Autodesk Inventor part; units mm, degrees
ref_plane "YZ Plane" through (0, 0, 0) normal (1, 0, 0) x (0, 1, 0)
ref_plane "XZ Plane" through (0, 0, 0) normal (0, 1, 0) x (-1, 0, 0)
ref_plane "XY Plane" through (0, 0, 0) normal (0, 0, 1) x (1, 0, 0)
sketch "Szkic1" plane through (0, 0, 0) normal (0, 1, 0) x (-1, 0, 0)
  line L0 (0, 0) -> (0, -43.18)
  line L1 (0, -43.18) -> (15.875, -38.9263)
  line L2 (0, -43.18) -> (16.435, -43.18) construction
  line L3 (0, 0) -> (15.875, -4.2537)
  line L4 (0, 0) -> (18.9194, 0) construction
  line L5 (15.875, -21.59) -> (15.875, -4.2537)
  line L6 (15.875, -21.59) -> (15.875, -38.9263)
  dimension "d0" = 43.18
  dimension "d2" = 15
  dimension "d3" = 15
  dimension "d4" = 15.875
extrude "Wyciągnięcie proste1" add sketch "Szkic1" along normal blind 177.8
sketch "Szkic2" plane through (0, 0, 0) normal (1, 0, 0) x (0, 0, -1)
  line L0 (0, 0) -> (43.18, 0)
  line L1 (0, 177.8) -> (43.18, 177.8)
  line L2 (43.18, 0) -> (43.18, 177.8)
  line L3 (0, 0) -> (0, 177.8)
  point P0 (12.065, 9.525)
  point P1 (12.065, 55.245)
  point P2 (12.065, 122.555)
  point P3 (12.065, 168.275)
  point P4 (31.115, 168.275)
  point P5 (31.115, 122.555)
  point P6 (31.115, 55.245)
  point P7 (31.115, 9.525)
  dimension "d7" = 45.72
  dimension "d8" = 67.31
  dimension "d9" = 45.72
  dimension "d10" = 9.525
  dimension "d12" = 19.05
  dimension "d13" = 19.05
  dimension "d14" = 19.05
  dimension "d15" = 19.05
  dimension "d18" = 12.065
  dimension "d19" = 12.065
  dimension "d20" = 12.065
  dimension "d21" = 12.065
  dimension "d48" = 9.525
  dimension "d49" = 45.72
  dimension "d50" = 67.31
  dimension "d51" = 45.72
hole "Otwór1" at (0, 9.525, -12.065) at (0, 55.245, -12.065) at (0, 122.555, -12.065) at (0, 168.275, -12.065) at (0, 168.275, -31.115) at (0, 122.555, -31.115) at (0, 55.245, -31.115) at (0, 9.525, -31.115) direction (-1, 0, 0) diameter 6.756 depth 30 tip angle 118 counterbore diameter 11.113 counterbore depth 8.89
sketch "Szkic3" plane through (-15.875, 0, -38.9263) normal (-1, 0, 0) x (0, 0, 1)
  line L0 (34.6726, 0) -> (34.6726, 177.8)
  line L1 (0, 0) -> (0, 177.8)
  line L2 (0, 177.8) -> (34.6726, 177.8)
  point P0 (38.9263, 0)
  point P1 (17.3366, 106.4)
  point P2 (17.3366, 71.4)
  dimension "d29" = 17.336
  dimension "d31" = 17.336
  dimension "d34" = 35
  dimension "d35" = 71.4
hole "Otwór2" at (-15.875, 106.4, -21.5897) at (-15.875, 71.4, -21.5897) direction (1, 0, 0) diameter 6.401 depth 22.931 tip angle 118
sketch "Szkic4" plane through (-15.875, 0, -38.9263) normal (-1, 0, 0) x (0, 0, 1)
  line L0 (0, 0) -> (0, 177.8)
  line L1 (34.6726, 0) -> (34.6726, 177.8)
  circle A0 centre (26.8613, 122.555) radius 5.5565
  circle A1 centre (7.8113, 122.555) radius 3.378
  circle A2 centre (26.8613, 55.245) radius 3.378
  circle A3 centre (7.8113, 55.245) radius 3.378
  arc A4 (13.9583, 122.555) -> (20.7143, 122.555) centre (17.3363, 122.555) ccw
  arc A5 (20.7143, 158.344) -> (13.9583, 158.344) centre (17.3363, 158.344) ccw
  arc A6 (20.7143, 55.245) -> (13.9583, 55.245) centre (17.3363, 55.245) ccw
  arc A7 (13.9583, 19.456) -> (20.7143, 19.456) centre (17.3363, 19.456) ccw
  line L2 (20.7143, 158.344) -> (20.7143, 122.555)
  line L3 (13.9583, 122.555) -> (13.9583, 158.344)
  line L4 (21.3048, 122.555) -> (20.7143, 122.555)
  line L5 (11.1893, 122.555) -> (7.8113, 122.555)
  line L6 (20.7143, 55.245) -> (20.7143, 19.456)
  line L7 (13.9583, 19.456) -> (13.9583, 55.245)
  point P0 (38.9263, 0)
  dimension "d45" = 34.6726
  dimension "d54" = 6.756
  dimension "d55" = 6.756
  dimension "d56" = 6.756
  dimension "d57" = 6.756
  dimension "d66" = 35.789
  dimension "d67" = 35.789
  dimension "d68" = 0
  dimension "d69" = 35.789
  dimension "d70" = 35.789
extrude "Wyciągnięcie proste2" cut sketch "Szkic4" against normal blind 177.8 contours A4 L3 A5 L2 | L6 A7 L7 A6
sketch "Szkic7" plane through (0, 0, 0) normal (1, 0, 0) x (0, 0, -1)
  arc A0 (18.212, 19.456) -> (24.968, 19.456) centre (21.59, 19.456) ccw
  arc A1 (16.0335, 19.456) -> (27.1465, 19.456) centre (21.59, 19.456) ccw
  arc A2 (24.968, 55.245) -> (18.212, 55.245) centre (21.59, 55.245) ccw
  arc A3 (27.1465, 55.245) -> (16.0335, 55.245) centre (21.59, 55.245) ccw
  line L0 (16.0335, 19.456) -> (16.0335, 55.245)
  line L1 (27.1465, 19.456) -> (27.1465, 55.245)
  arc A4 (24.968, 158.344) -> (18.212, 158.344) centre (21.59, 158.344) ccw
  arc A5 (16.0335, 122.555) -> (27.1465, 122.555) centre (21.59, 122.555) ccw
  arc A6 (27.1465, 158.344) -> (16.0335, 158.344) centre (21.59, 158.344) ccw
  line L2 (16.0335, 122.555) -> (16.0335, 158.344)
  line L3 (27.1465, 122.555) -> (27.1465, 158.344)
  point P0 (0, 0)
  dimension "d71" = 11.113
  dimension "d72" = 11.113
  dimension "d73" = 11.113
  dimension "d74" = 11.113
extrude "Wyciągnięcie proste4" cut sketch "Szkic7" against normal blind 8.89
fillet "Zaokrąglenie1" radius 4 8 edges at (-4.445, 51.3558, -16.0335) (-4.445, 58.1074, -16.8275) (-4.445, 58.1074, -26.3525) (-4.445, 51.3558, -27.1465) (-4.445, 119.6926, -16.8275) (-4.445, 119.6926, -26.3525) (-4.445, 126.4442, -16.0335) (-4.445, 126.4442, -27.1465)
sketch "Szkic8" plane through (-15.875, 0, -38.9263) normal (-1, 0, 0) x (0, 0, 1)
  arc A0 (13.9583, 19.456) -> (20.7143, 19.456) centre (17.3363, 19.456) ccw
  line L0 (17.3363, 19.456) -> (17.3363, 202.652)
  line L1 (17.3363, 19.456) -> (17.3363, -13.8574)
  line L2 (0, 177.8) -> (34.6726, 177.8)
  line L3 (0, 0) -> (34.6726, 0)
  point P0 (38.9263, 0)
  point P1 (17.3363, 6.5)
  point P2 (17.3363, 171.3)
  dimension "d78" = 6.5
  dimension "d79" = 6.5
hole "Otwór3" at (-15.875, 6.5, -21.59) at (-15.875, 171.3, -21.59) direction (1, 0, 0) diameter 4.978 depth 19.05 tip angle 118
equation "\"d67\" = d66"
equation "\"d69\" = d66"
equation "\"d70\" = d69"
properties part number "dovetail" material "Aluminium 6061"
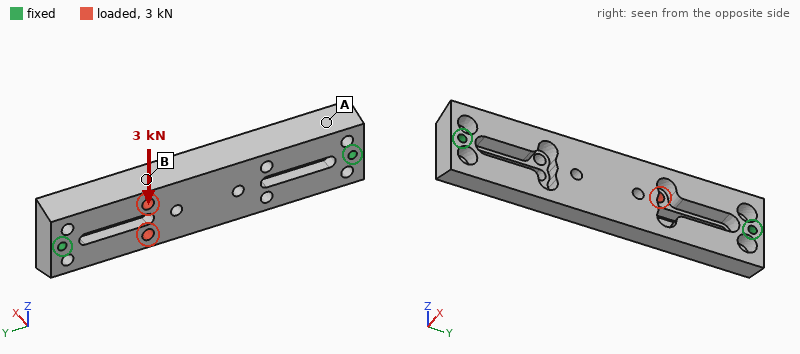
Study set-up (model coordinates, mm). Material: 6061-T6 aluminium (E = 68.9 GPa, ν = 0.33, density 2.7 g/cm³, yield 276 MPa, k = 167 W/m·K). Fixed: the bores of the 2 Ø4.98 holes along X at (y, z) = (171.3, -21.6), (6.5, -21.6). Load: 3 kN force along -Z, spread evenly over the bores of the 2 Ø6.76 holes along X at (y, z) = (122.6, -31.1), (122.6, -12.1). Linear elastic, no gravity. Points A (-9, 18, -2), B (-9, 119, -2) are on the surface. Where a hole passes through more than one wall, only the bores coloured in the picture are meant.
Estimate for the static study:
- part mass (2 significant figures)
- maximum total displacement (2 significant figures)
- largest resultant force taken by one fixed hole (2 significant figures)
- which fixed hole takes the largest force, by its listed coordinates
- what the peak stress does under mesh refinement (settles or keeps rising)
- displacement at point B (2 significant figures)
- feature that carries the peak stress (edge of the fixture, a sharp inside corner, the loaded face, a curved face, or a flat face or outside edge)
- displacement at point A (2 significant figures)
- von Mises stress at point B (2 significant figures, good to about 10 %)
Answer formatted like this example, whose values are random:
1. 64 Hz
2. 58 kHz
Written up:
1. 230 g
2. 77 µm
3. 2.1 kN
4. (171.3, -21.6)
5. keeps rising
6. 71 µm
7. edge of the fixture
8. 15 µm
9. 45 MPa
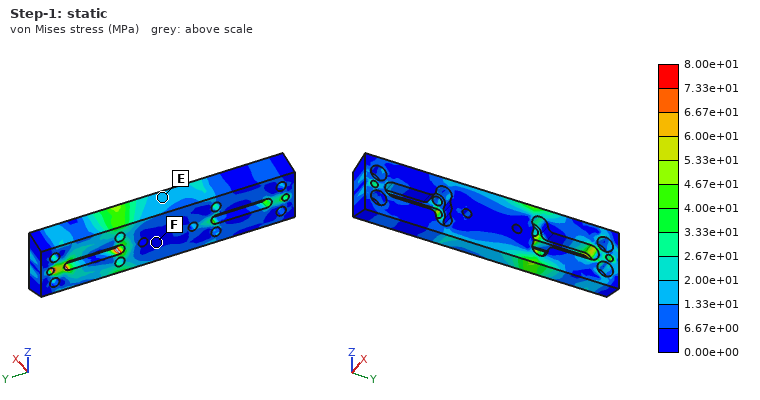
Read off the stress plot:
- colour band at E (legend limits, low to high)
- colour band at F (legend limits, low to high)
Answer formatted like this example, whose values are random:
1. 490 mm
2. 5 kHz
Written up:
1. 1.33e+01 to 2.00e+01 MPa
2. 0.00e+00 to 6.67e+00 MPa
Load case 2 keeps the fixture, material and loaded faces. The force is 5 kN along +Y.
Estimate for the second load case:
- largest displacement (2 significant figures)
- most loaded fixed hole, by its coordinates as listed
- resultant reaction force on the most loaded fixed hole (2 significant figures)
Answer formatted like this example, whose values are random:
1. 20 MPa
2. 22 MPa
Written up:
1. 17 µm
2. (171.3, -21.6)
3. 3.2 kN
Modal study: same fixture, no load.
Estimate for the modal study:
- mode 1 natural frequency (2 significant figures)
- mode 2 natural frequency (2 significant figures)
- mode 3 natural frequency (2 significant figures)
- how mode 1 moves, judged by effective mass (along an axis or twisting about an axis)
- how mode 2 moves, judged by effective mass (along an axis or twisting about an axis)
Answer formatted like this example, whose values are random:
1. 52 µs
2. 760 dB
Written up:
1. 2100 Hz
2. 2700 Hz
3. 3800 Hz
4. along X
5. along Z
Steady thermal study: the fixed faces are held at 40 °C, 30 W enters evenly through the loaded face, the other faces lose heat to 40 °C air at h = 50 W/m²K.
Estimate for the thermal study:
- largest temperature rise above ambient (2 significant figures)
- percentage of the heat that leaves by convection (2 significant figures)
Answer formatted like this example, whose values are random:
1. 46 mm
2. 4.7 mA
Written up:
1. 15 K
2. 26 %
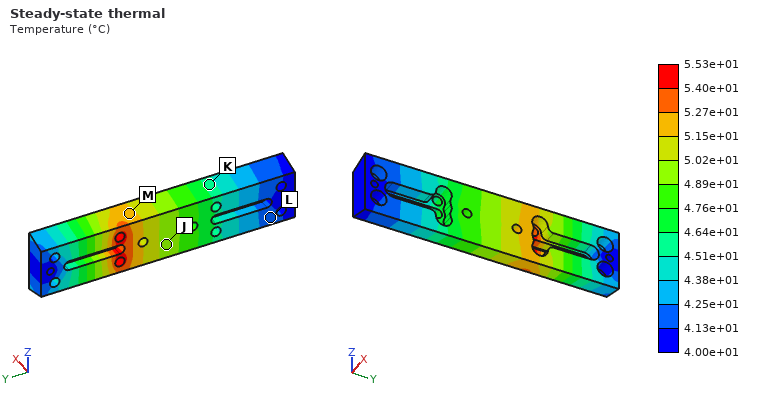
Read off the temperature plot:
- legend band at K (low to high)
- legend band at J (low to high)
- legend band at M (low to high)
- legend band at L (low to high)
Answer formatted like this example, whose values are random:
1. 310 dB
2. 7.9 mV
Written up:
1. 4.51e+01 to 4.64e+01 °C
2. 4.89e+01 to 5.02e+01 °C
3. 5.15e+01 to 5.27e+01 °C
4. 4.13e+01 to 4.25e+01 °C
